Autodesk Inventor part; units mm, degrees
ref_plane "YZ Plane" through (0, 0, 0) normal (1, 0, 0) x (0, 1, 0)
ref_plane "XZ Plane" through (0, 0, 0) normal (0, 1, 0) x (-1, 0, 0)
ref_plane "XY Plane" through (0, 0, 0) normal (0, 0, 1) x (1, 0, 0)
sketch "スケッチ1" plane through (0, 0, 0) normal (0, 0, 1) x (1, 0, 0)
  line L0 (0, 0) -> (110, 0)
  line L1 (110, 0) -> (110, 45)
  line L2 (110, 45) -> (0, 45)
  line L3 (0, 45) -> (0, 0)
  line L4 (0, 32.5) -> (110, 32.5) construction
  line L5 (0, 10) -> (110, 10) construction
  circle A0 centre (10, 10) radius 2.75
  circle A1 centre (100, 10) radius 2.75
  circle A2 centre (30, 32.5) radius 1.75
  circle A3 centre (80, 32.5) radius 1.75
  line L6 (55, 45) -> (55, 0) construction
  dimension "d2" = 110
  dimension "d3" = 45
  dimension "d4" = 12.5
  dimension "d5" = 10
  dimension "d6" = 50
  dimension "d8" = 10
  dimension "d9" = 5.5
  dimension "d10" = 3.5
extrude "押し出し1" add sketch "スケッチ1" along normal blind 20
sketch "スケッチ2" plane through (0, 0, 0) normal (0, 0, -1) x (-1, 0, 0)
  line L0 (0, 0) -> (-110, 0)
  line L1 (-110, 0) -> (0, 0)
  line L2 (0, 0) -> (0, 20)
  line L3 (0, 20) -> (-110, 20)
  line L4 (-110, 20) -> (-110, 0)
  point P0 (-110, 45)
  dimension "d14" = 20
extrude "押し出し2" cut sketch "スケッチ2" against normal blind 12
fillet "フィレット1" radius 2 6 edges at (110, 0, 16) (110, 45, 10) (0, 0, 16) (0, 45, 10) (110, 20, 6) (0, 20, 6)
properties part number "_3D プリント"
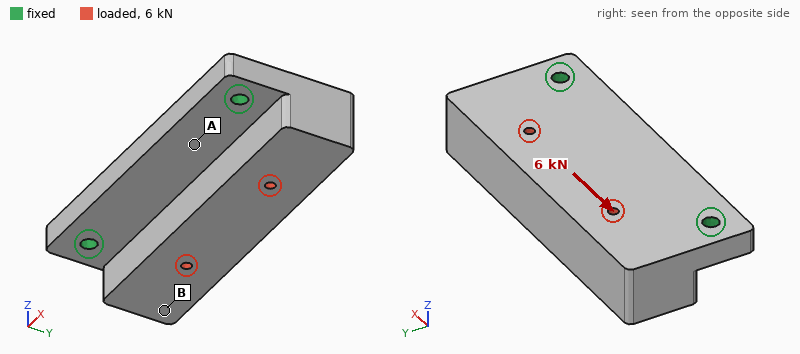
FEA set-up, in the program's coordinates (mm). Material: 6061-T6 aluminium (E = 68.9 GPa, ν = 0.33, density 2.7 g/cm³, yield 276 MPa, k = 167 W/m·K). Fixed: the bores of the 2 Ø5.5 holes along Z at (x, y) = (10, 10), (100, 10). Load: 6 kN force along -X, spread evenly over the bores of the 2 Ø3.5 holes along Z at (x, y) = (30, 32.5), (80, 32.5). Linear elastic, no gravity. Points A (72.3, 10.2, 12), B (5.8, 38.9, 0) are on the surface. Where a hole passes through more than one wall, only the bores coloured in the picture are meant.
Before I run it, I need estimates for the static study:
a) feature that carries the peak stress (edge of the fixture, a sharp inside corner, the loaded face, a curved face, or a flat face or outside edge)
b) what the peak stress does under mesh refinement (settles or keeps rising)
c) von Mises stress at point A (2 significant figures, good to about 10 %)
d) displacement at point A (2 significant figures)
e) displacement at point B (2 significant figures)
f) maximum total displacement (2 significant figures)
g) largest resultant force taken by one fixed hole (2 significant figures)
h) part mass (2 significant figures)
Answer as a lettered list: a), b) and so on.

a) edge of the fixture
b) keeps rising
c) 8.6 MPa
d) 4.9 µm
e) 11 µm
f) 12 µm
g) 3.3 kN
h) 190 g
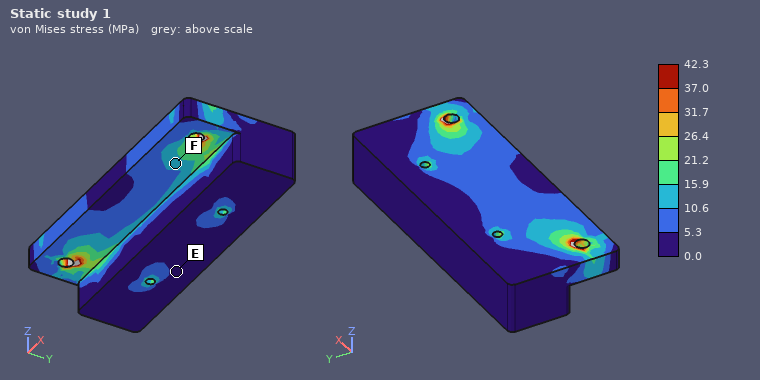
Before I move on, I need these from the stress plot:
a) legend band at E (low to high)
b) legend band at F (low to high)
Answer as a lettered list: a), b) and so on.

a) 0.0 to 5.3 MPa
b) 10.6 to 15.9 MPa
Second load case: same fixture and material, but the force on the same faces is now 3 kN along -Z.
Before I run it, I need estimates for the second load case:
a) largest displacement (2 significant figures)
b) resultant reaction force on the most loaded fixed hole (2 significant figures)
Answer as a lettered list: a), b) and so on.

a) 0.16 mm
b) 1.5 kN
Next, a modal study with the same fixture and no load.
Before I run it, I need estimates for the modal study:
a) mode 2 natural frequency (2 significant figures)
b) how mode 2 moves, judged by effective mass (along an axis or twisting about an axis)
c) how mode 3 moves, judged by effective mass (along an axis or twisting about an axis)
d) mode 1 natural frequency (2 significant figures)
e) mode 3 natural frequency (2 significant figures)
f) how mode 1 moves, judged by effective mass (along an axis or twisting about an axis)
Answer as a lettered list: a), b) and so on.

a) 6000 Hz
b) twisting about Y
c) along Z
d) 2200 Hz
e) 6400 Hz
f) along Z
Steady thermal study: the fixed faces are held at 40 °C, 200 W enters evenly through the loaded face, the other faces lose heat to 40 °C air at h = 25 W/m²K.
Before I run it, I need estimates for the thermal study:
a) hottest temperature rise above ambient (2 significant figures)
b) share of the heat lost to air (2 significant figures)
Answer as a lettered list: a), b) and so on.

a) 56 K
b) 7.1 %
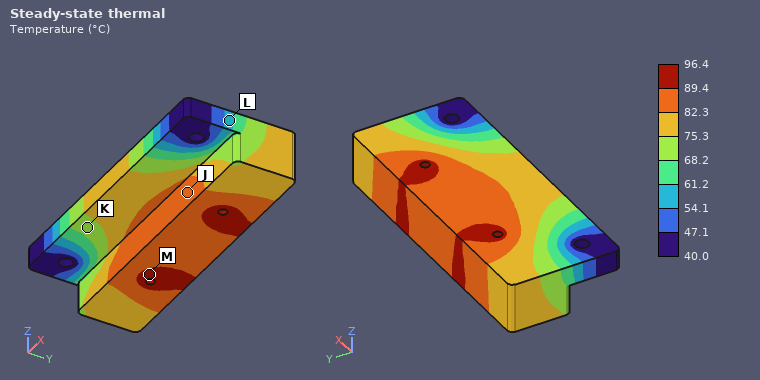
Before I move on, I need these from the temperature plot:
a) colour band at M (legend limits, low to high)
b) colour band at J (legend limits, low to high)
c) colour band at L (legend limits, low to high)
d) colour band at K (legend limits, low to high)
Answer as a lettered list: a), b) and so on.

a) 89.4 to 96.4 °C
b) 82.3 to 89.4 °C
c) 54.1 to 61.2 °C
d) 68.2 to 75.3 °C
